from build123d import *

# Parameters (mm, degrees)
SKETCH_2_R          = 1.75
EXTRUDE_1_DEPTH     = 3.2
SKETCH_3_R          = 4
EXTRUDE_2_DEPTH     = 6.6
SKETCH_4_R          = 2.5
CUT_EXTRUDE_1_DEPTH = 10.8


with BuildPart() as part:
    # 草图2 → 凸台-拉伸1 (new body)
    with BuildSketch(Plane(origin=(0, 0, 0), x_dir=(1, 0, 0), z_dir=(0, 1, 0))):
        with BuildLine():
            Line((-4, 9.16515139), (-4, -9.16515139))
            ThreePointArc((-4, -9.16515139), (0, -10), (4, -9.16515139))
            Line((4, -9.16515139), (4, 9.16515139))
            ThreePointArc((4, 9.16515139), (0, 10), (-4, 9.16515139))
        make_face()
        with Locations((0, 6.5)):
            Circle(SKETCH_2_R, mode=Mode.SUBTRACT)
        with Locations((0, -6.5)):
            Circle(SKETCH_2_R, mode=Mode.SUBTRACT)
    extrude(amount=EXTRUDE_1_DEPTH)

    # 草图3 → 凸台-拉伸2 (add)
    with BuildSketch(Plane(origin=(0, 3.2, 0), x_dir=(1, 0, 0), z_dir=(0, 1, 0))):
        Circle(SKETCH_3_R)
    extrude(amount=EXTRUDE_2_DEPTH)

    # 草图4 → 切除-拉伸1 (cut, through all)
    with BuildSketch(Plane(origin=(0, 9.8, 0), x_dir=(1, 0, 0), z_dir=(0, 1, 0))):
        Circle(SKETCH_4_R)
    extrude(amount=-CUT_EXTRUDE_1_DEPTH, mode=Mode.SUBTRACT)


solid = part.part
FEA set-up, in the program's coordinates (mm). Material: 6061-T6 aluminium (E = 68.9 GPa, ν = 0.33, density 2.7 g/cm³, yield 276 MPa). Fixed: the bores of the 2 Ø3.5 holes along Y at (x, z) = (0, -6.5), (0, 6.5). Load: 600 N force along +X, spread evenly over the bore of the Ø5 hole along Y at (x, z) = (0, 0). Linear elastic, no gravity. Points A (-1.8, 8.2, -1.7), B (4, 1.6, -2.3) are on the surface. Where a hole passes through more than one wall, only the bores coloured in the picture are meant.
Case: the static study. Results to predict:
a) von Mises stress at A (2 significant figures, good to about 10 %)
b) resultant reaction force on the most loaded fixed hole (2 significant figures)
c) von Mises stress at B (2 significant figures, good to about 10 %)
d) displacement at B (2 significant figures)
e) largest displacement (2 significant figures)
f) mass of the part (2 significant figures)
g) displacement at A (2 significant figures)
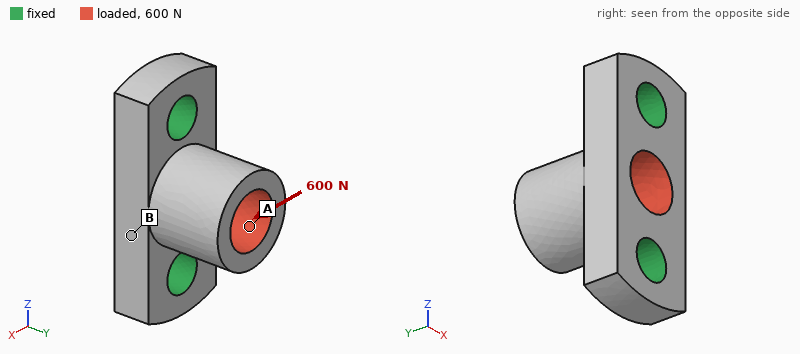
14 MPa
300 N
38 MPa
5.4 µm
20 µm
1.6 g
15 µm
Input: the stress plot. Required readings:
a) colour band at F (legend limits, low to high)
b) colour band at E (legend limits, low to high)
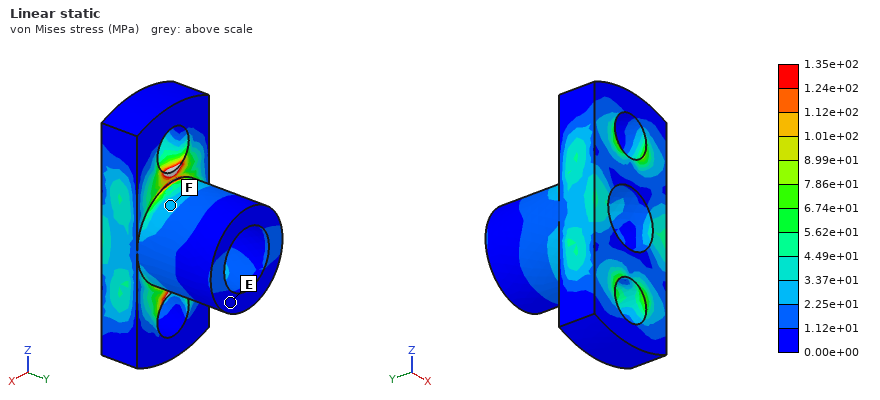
2.25e+01 to 3.37e+01 MPa
0.00e+00 to 1.12e+01 MPa
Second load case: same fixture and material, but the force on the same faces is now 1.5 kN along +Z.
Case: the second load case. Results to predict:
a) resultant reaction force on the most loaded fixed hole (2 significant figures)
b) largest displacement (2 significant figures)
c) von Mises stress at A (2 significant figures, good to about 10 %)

910 N
19 µm
37 MPa
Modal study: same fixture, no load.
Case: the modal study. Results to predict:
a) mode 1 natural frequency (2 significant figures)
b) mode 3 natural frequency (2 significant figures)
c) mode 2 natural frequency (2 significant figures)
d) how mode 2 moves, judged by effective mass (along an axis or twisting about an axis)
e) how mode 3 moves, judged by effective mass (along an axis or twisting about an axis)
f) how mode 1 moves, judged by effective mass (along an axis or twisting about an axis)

35 kHz
76 kHz
59 kHz
along Z
along Y
along X
